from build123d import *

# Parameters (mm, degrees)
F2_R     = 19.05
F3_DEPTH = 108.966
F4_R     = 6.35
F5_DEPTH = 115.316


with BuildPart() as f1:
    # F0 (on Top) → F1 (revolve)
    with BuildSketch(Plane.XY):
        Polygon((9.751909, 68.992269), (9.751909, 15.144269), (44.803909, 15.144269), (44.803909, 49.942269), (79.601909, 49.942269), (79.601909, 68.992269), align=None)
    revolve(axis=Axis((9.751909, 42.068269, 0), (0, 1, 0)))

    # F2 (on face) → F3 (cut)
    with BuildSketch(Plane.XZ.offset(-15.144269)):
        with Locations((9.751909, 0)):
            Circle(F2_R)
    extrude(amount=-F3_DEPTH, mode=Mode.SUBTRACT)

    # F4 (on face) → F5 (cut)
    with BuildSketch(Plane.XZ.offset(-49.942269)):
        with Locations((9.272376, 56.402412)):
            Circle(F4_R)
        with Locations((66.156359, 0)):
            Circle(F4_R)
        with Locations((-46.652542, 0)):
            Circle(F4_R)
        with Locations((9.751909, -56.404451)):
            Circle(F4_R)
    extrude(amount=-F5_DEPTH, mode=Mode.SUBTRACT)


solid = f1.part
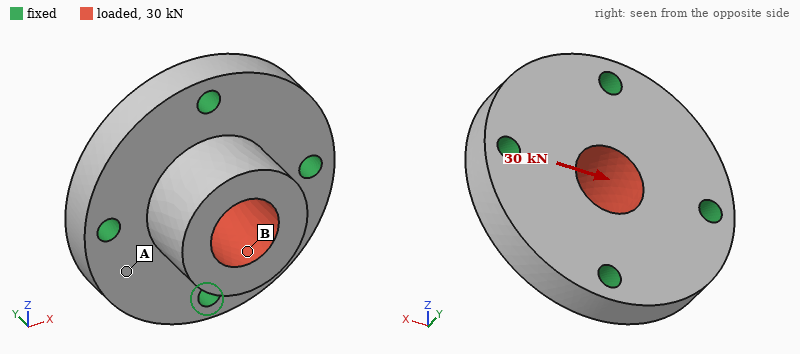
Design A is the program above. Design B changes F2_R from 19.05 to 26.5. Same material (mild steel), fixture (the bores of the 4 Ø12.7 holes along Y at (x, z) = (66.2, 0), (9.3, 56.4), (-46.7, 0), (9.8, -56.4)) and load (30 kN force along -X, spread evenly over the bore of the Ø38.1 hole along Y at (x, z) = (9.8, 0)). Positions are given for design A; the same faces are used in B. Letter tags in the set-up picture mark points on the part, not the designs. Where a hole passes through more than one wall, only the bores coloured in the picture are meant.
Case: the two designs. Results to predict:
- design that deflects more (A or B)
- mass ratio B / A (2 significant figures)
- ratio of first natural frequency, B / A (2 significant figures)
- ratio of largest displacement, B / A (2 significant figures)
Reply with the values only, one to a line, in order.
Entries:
B
0.84
1.0
1.4
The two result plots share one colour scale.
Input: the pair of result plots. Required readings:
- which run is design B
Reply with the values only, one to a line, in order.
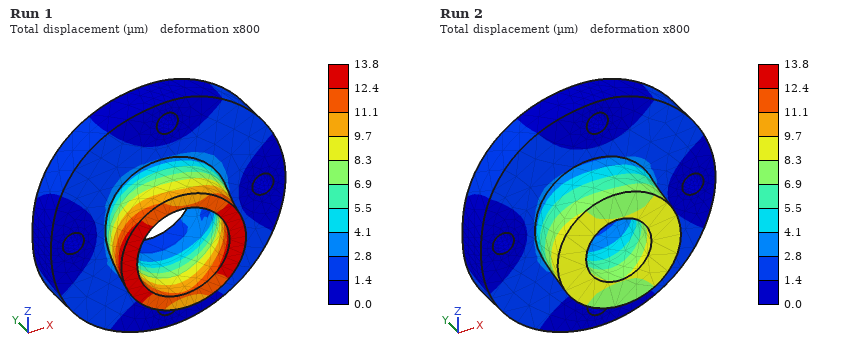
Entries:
Run 1
